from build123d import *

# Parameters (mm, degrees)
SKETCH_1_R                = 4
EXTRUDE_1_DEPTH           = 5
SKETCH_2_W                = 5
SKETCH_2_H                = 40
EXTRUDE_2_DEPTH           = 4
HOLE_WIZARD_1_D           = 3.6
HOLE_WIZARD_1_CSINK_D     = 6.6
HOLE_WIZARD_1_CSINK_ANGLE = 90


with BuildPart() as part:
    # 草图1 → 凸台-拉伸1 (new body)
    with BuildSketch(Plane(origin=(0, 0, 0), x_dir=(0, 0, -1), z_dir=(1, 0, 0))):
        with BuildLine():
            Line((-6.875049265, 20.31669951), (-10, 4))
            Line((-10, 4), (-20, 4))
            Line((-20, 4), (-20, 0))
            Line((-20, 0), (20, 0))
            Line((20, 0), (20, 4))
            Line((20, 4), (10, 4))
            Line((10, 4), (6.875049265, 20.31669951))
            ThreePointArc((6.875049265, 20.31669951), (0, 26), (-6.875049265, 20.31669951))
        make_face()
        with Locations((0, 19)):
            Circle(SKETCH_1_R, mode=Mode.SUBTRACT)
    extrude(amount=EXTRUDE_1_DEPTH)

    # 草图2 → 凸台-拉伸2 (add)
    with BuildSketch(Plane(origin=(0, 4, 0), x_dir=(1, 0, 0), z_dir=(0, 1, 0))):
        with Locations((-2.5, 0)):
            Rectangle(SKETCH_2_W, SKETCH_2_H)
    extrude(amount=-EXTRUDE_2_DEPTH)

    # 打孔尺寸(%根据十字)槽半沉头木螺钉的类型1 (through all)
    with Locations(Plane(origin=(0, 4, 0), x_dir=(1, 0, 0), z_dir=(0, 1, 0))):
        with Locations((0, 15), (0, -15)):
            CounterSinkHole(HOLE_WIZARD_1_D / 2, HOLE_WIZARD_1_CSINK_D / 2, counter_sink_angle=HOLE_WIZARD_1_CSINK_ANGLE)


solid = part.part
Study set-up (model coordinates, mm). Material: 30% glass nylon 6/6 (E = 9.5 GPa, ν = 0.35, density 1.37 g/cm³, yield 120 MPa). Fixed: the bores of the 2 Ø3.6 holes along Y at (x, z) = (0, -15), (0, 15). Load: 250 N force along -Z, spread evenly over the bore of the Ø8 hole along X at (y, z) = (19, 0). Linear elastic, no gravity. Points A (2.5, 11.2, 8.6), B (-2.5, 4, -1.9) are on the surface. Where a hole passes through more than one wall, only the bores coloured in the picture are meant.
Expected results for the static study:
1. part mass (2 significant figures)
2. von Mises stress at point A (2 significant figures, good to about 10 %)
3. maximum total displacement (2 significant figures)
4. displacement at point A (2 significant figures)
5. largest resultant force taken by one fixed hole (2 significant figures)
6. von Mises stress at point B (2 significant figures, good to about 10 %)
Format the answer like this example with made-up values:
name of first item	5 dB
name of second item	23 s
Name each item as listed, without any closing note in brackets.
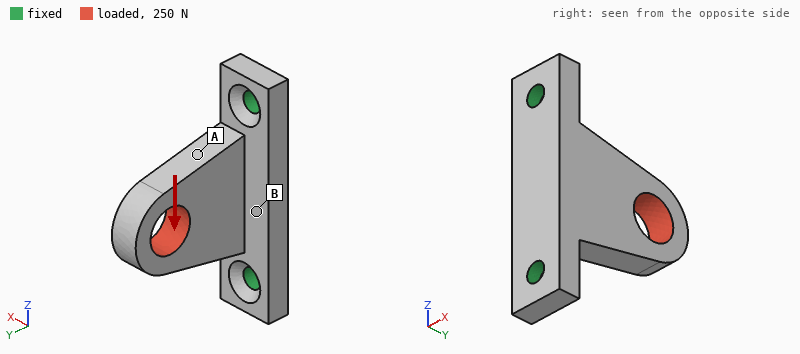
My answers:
part mass	4.0 g
von Mises stress at point A	11 MPa
maximum total displacement	0.11 mm
displacement at point A	0.040 mm
largest resultant force taken by one fixed hole	220 N
von Mises stress at point B	4.8 MPa
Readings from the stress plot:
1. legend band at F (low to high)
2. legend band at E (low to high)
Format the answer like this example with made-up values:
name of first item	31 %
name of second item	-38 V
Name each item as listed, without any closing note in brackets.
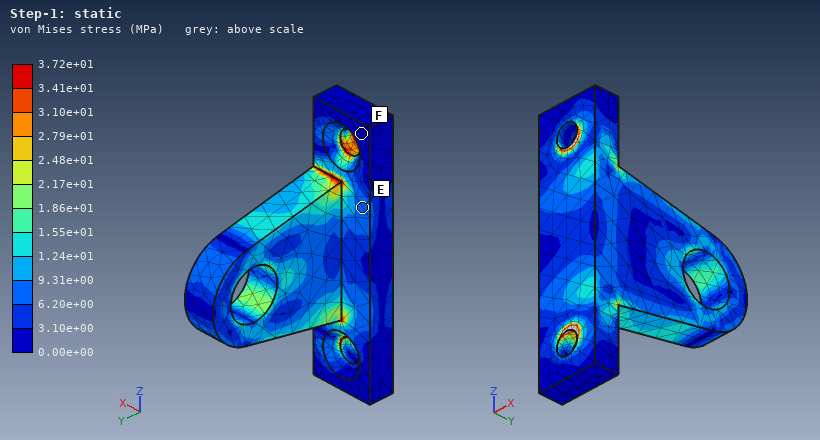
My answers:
legend band at F	0.00e+00 to 3.10e+00 MPa
legend band at E	6.20e+00 to 9.31e+00 MPa
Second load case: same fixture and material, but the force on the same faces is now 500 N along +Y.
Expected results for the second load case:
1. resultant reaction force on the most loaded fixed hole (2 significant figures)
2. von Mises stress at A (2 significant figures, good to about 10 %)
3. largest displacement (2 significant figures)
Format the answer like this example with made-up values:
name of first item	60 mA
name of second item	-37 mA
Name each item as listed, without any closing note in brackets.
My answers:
resultant reaction force on the most loaded fixed hole	300 N
von Mises stress at A	10 MPa
largest displacement	0.19 mm
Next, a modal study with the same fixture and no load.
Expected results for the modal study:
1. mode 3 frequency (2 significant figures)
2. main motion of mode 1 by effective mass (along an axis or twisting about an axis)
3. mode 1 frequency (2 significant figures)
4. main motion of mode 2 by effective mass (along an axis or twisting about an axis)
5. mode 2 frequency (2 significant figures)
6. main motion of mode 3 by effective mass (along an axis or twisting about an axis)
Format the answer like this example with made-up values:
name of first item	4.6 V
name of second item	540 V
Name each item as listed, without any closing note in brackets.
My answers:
mode 3 frequency	9600 Hz
main motion of mode 1 by effective mass	along X
mode 1 frequency	2800 Hz
main motion of mode 2 by effective mass	along Z
mode 2 frequency	9000 Hz
main motion of mode 3 by effective mass	along Y
